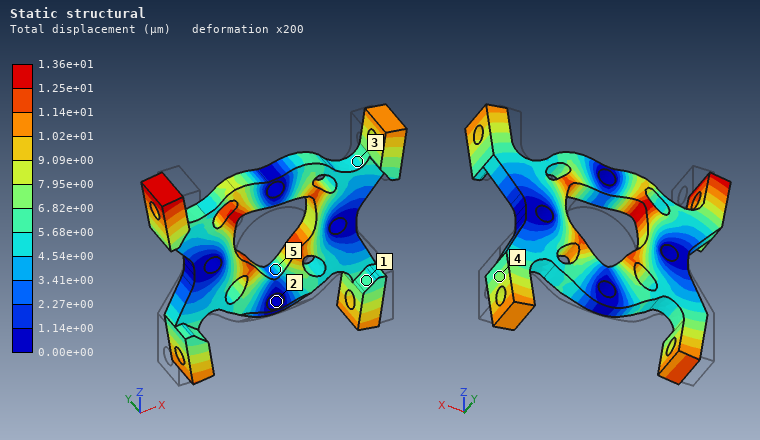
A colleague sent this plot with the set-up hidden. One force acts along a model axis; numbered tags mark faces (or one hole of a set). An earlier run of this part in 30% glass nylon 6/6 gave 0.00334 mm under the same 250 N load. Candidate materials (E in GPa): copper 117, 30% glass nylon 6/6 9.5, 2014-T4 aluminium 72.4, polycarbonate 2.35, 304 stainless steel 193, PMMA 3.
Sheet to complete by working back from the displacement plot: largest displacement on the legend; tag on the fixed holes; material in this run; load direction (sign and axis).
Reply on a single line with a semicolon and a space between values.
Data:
1.36e+01 µm; 2; polycarbonate; +Z
